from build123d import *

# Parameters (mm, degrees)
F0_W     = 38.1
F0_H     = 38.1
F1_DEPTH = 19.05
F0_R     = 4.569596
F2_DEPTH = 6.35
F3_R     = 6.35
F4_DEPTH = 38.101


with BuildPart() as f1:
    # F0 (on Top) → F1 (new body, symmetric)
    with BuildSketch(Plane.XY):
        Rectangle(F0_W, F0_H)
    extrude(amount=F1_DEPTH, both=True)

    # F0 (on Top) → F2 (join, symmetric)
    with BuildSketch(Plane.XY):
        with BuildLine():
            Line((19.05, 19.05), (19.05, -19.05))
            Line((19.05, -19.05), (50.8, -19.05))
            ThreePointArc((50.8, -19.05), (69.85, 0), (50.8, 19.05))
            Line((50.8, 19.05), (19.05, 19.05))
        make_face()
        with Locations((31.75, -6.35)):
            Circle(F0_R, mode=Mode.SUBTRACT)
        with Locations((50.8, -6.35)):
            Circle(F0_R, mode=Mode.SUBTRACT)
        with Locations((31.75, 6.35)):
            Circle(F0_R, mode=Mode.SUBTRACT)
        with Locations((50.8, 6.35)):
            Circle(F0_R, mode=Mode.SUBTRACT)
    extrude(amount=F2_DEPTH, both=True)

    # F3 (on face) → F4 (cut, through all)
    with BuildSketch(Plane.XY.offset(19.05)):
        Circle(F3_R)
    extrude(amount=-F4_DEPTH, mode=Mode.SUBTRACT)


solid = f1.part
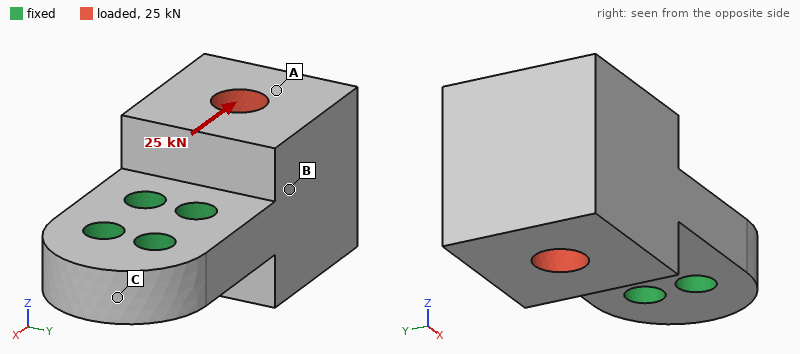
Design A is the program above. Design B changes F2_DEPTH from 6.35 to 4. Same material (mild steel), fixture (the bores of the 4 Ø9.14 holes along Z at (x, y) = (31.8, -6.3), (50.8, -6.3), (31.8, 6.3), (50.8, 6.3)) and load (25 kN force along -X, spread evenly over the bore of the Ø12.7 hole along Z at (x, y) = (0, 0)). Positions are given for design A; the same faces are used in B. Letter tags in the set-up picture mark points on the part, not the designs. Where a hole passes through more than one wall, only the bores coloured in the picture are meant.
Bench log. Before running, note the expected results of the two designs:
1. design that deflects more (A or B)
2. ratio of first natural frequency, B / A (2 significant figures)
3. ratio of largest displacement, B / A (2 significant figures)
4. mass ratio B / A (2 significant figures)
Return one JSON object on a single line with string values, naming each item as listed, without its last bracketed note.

{"design that deflects more": "B", "ratio of first natural frequency, B / A": "0.54", "ratio of largest displacement, B / A": "1.3", "mass ratio B / A": "0.90"}
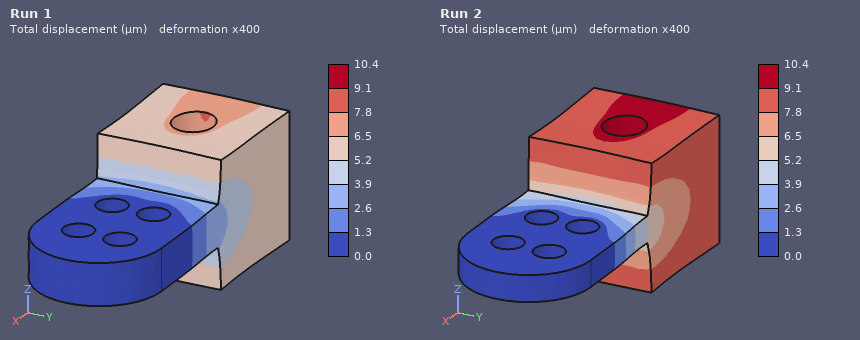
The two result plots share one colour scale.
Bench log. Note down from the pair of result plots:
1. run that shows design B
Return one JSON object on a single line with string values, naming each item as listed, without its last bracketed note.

{"run that shows design B": "Run 2"}
